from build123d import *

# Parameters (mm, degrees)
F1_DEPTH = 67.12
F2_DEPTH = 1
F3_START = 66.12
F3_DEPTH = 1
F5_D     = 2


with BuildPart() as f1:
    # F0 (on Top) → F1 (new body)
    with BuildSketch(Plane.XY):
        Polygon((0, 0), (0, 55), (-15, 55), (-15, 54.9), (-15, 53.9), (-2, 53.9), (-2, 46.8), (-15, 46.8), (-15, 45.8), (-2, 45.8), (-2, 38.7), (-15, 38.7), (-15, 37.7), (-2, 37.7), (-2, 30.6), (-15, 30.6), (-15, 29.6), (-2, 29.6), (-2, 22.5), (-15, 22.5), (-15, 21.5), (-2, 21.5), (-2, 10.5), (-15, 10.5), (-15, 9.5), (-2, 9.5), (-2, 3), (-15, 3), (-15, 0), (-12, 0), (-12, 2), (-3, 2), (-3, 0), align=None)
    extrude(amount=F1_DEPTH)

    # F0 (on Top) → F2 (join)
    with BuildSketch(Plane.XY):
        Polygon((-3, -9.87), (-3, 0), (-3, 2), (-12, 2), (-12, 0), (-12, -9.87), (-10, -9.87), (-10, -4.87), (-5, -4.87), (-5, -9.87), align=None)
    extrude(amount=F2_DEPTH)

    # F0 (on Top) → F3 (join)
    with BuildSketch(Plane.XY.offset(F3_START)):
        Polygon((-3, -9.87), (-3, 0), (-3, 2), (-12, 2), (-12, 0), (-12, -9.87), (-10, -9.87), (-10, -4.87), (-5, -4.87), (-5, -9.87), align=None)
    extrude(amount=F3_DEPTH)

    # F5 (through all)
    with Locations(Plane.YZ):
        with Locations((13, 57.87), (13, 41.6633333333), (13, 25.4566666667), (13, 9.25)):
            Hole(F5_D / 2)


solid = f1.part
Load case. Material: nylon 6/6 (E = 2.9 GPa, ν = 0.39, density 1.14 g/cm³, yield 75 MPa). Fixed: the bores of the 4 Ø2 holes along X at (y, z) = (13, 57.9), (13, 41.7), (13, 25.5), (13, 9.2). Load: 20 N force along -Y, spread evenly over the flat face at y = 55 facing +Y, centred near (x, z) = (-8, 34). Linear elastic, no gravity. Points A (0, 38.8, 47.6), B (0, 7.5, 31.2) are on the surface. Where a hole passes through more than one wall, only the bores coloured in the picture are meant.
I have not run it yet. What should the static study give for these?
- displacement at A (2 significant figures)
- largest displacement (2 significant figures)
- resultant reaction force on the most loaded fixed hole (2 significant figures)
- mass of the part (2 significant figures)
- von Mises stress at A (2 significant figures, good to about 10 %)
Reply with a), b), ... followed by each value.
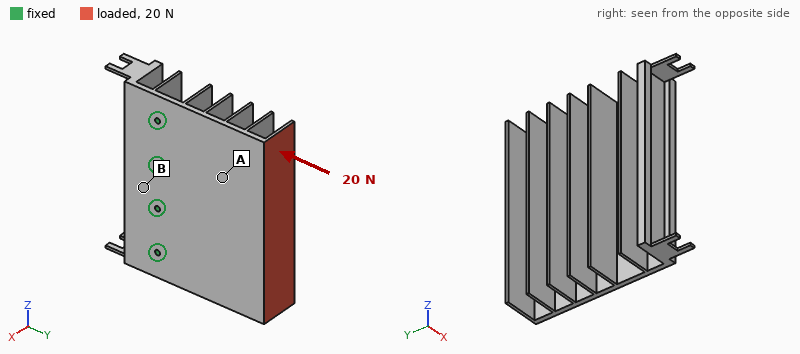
a) 0.31 mm
b) 1.1 mm
c) 5.3 N
d) 16 g
e) 2.2 MPa
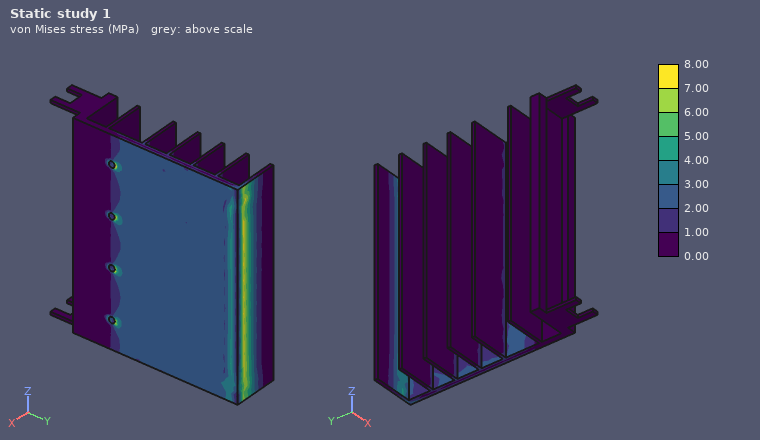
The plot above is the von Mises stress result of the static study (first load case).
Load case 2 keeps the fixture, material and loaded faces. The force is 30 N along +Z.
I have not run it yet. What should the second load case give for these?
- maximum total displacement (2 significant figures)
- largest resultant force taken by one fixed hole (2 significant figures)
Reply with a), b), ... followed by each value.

a) 0.87 mm
b) 25 N
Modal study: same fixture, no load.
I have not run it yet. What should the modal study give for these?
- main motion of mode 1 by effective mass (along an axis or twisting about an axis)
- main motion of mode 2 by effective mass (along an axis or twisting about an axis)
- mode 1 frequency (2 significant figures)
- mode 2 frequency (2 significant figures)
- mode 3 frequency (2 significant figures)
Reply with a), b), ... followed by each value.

a) along X
b) twisting about Y
c) 200 Hz
d) 350 Hz
e) 880 Hz
